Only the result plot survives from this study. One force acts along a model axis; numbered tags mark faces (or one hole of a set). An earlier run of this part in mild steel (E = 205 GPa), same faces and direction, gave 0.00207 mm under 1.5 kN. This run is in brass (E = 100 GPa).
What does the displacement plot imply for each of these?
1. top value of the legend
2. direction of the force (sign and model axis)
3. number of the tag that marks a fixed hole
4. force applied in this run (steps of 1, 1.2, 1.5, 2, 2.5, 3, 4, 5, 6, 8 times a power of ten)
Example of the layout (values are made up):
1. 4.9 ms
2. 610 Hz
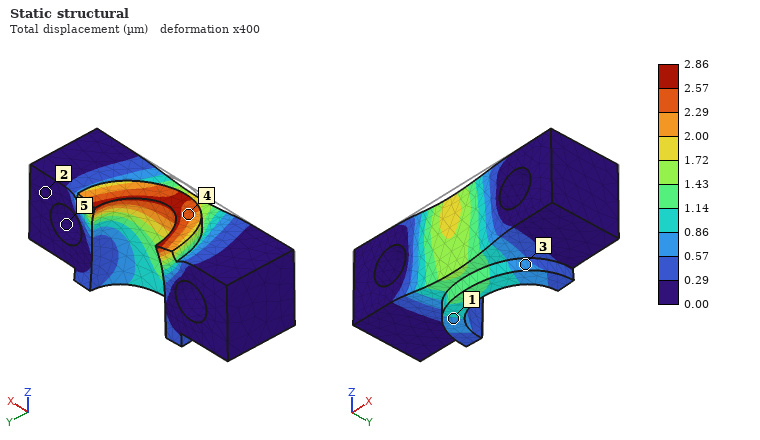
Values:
1. 2.86 µm
2. -Z
3. 5
4. 1 kN
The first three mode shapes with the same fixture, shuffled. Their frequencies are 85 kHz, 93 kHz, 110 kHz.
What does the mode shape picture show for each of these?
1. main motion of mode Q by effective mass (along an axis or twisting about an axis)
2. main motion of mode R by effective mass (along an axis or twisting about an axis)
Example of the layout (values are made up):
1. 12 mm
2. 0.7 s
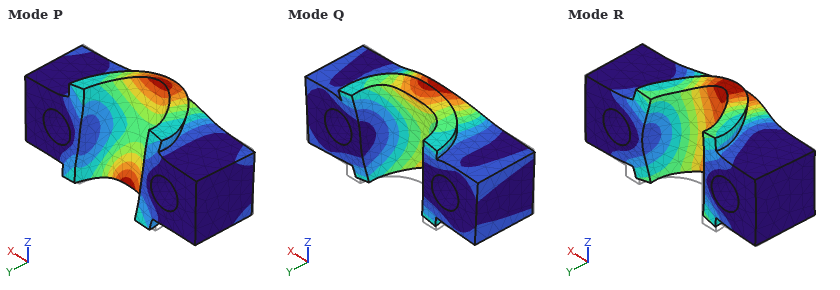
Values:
1. along Z
2. along Y
